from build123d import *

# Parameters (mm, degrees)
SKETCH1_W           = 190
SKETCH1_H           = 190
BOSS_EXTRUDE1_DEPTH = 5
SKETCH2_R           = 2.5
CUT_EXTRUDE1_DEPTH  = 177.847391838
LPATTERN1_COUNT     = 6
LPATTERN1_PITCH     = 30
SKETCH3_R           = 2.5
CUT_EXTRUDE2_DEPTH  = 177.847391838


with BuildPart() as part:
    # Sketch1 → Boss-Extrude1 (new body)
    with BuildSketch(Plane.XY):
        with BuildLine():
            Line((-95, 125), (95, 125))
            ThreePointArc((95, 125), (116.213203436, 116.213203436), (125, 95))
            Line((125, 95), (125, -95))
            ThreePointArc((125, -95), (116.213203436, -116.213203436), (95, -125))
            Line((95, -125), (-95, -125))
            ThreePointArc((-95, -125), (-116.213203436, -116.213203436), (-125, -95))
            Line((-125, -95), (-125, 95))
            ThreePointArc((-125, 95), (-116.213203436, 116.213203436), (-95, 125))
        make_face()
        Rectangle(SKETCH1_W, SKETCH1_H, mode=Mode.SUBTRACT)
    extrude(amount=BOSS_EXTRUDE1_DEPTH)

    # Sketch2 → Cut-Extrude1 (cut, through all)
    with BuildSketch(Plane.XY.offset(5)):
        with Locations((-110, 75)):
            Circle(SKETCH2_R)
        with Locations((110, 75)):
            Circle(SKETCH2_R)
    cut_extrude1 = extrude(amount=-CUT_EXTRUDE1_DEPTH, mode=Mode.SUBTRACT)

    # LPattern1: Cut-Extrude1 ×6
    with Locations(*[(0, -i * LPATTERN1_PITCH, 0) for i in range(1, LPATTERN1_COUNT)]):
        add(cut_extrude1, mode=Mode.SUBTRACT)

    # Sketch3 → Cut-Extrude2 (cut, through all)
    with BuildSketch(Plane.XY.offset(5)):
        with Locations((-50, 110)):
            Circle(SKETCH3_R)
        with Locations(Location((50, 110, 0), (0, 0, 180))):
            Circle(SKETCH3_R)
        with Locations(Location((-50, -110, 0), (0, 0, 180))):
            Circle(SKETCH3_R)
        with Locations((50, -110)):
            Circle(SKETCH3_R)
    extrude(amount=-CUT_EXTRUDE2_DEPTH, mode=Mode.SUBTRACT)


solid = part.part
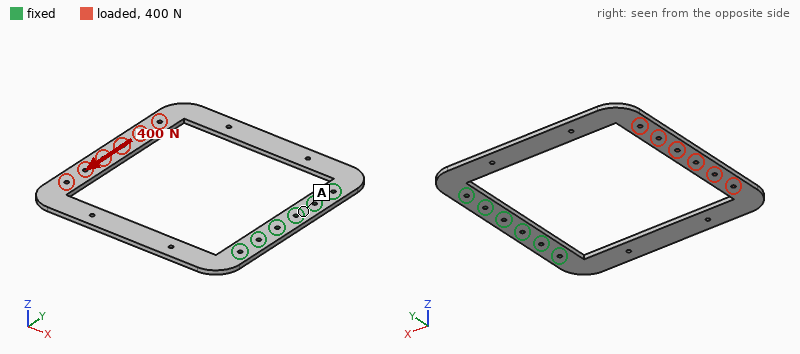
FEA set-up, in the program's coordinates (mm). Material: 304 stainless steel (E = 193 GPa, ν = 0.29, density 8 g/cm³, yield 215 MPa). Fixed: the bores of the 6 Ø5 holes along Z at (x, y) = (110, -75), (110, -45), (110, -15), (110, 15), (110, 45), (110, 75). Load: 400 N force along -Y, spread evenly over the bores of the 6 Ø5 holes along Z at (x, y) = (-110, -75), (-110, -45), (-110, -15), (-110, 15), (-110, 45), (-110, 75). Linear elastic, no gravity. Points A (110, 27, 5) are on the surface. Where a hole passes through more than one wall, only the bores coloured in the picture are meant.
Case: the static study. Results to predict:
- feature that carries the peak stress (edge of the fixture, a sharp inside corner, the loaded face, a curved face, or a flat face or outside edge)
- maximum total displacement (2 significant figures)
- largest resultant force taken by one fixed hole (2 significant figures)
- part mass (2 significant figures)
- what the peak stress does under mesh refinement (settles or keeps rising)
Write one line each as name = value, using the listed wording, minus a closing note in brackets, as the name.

feature that carries the peak stress = edge of the fixture
maximum total displacement = 0.20 mm
largest resultant force taken by one fixed hole = 910 N
part mass = 1.0 kg
what the peak stress does under mesh refinement = keeps rising
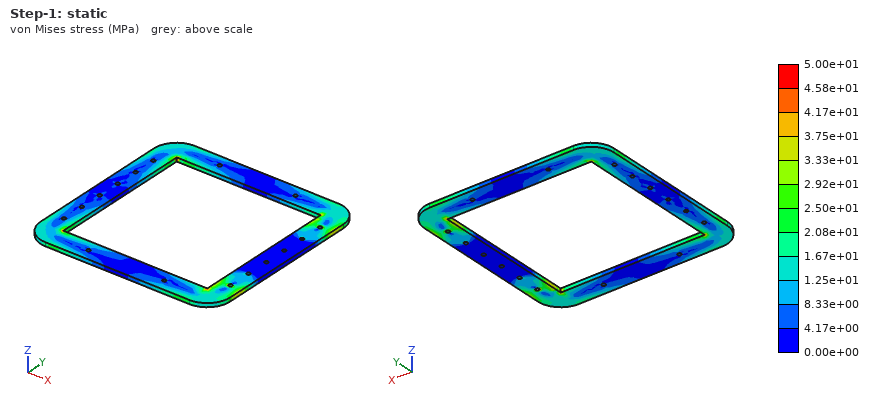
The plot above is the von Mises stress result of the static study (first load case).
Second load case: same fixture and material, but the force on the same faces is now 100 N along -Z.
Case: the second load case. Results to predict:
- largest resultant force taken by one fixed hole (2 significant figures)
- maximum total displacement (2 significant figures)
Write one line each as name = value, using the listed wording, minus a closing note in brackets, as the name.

largest resultant force taken by one fixed hole = 62 N
maximum total displacement = 4.0 mm
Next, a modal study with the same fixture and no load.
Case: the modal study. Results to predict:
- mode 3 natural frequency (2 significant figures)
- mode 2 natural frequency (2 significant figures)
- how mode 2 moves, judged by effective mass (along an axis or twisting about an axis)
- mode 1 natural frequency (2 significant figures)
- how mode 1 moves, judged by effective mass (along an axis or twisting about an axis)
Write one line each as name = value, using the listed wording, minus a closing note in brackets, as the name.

mode 3 natural frequency = 290 Hz
mode 2 natural frequency = 100 Hz
how mode 2 moves, judged by effective mass = twisting about X
mode 1 natural frequency = 43 Hz
how mode 1 moves, judged by effective mass = along Z
